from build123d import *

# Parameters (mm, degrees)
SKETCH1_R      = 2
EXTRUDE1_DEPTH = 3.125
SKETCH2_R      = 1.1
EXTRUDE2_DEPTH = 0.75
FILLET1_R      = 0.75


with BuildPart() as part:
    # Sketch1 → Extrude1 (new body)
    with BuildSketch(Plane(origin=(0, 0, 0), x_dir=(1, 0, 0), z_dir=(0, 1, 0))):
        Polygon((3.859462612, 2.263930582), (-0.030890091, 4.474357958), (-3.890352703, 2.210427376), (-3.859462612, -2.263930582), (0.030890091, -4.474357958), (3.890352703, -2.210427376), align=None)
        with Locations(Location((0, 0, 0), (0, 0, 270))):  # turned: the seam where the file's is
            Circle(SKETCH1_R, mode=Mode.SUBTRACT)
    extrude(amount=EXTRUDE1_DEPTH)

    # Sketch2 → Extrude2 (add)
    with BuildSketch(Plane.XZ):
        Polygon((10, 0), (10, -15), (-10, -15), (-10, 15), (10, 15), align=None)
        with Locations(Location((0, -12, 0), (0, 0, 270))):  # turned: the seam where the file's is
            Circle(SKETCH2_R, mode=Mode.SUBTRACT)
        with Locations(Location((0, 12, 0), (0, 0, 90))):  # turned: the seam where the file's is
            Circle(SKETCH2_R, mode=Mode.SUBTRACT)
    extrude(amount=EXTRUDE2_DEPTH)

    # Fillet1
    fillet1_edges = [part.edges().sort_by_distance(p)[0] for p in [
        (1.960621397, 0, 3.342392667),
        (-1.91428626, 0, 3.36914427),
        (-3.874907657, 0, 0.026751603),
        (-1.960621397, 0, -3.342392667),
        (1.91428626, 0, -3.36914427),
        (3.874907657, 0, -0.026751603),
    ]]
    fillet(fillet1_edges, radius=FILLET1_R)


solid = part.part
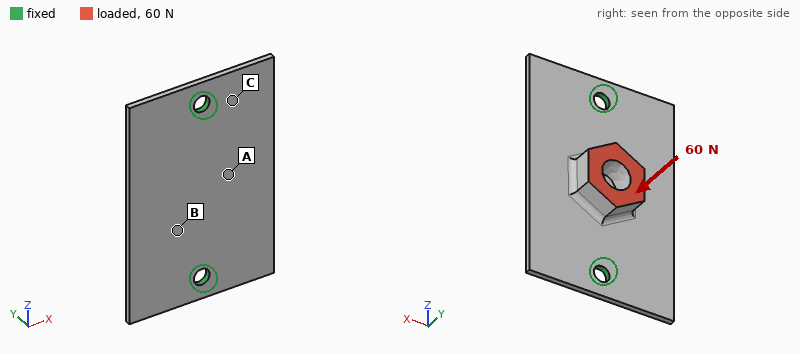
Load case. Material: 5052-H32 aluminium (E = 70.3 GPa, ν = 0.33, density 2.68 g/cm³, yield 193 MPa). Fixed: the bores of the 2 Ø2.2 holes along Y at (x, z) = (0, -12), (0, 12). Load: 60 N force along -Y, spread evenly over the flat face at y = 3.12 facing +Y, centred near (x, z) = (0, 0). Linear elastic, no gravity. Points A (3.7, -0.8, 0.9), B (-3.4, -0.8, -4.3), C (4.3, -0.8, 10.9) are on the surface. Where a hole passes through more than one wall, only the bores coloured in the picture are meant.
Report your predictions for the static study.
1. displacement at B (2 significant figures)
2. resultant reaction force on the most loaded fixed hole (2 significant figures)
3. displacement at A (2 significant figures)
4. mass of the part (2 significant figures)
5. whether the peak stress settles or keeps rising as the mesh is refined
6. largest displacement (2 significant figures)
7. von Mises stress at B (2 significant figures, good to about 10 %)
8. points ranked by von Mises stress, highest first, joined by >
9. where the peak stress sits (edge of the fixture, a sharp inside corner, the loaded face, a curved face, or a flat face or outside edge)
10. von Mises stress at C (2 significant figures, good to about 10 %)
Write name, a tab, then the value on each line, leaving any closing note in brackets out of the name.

displacement at B	43 µm
resultant reaction force on the most loaded fixed hole	35 N
displacement at A	47 µm
mass of the part	1.5 g
whether the peak stress settles or keeps rising as the mesh is refined	keeps rising
largest displacement	50 µm
von Mises stress at B	45 MPa
points ranked by von Mises stress, highest first, joined by >	B > C > A
where the peak stress sits	edge of the fixture
von Mises stress at C	29 MPa
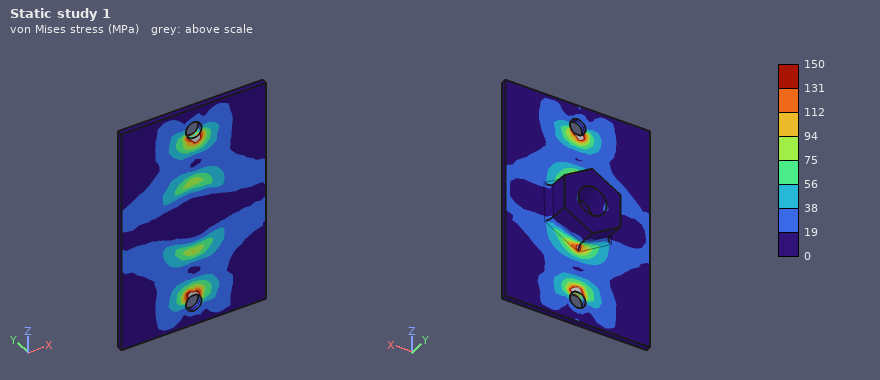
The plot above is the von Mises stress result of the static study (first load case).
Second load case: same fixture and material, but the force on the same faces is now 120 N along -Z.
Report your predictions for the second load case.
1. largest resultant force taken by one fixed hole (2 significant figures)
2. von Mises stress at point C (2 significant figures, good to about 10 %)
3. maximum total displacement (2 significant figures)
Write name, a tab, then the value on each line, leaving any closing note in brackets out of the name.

largest resultant force taken by one fixed hole	65 N
von Mises stress at point C	15 MPa
maximum total displacement	26 µm
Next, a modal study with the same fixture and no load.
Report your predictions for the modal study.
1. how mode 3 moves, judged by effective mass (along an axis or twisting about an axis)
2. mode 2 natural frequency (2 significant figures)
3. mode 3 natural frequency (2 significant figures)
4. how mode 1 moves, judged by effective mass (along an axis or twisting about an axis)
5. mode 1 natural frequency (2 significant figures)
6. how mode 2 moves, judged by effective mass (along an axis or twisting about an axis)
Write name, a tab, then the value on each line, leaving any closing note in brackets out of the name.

how mode 3 moves, judged by effective mass	twisting about X
mode 2 natural frequency	5800 Hz
mode 3 natural frequency	9000 Hz
how mode 1 moves, judged by effective mass	twisting about Z
mode 1 natural frequency	4200 Hz
how mode 2 moves, judged by effective mass	along Y
